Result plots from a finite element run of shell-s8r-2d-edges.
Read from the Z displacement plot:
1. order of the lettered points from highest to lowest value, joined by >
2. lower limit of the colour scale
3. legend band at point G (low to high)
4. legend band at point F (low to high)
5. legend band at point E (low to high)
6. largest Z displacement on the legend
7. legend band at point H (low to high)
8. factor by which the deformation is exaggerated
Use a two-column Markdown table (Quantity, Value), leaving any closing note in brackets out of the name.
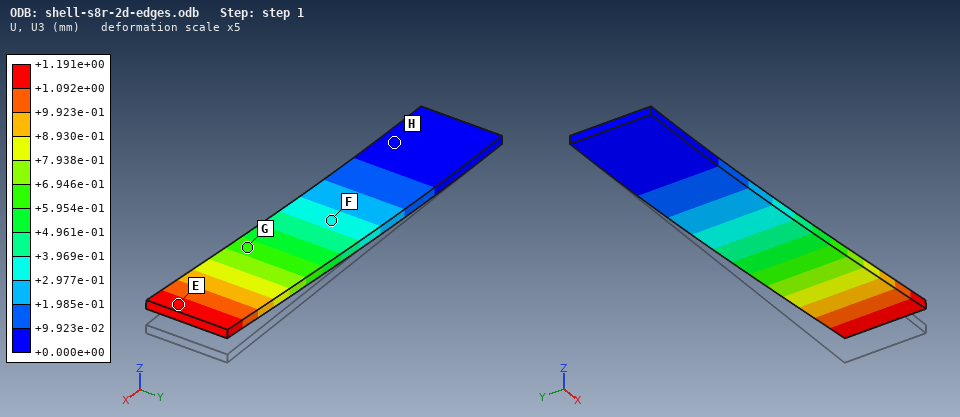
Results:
| Quantity | Value |
|---|---|
| order of the lettered points from highest to lowest value, joined by > | E > G > F > H |
| lower limit of the colour scale | +0.000e+00 mm |
| legend band at point G | +5.954e-01 to +6.946e-01 mm |
| legend band at point F | +2.977e-01 to +3.969e-01 mm |
| legend band at point E | +1.092e+00 to +1.191e+00 mm |
| largest Z displacement on the legend | +1.191e+00 mm |
| legend band at point H | +0.000e+00 to +9.923e-02 mm |
| factor by which the deformation is exaggerated | 5 |
